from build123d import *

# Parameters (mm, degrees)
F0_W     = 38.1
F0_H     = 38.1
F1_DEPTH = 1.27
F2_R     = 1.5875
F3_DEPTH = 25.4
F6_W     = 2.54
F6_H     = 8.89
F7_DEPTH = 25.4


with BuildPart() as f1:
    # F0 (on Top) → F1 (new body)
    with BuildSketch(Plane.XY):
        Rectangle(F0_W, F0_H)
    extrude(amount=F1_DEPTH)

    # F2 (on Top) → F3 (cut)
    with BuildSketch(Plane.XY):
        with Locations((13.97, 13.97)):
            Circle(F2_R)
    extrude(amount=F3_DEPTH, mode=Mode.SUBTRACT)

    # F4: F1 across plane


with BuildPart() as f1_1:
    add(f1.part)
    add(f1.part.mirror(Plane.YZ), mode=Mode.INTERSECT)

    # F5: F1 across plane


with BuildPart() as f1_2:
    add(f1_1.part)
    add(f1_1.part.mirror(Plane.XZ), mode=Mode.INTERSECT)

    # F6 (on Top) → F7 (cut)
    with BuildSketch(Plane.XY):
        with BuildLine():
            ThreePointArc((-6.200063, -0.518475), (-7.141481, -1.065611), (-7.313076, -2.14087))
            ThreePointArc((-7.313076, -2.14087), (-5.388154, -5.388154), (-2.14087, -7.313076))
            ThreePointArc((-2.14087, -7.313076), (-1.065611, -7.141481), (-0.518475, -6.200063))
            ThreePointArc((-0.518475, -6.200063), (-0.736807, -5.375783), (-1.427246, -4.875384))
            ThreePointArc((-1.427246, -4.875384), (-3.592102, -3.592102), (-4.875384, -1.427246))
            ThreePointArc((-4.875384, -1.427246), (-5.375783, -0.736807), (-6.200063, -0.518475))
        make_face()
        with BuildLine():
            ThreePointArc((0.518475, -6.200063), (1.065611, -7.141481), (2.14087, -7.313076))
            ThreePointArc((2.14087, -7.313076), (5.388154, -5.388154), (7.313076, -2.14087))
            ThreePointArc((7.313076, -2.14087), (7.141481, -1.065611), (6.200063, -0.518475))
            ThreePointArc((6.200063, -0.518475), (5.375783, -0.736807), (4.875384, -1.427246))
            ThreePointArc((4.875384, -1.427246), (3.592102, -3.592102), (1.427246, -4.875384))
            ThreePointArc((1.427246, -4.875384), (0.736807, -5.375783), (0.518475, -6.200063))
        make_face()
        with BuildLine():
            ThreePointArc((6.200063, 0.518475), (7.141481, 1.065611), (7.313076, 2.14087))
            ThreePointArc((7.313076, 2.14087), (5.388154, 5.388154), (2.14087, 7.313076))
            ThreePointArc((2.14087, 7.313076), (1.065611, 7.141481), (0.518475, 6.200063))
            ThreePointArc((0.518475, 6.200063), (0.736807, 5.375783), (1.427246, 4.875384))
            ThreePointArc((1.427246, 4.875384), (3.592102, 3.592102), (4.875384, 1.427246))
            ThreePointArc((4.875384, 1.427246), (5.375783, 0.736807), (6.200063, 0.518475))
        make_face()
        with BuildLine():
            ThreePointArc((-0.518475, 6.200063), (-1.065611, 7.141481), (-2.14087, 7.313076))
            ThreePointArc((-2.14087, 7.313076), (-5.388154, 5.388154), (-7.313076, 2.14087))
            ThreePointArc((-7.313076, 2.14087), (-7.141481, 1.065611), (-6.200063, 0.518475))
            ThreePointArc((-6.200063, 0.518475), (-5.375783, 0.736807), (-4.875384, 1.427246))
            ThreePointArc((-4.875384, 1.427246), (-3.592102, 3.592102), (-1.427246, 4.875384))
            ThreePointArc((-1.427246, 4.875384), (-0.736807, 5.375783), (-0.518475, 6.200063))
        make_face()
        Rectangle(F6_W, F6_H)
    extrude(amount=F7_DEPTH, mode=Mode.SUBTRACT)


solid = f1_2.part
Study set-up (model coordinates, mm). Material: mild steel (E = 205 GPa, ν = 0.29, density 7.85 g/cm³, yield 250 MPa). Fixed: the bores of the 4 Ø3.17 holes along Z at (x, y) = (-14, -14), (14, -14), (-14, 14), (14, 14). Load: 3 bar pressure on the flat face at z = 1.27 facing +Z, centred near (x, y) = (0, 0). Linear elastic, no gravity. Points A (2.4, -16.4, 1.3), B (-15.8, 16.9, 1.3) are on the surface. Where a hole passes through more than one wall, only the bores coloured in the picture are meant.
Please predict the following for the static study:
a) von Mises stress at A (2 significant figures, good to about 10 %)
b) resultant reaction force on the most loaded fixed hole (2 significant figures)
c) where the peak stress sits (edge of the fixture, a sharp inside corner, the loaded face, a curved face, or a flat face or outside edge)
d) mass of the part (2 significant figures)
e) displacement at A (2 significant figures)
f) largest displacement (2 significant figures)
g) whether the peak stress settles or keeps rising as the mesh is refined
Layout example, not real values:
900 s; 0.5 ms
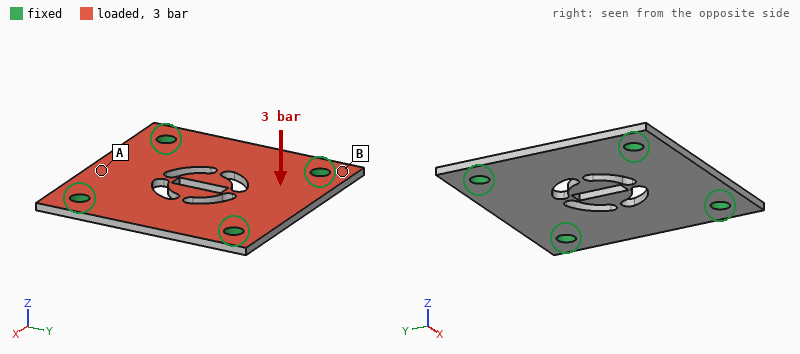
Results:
32 MPa; 98 N; edge of the fixture; 13 g; 10 µm; 29 µm; keeps rising
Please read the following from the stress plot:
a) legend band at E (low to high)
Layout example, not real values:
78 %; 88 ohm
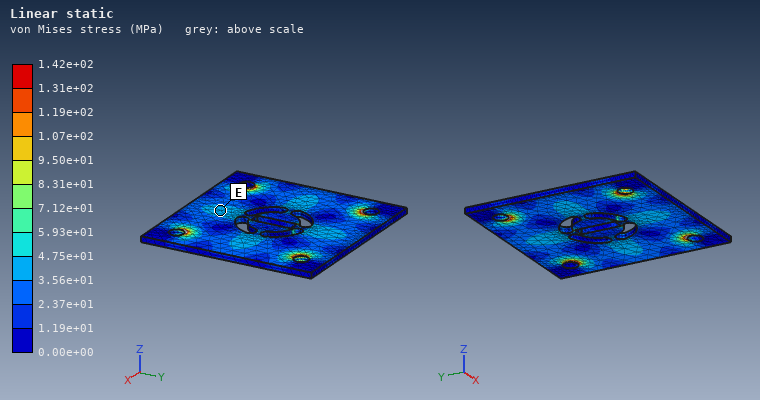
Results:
3.56e+01 to 4.75e+01 MPa
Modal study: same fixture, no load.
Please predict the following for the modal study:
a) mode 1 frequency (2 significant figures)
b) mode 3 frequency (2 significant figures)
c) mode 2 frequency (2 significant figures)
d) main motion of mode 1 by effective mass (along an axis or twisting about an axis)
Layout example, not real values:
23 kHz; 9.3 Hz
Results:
6700 Hz; 10000 Hz; 9900 Hz; along Z
